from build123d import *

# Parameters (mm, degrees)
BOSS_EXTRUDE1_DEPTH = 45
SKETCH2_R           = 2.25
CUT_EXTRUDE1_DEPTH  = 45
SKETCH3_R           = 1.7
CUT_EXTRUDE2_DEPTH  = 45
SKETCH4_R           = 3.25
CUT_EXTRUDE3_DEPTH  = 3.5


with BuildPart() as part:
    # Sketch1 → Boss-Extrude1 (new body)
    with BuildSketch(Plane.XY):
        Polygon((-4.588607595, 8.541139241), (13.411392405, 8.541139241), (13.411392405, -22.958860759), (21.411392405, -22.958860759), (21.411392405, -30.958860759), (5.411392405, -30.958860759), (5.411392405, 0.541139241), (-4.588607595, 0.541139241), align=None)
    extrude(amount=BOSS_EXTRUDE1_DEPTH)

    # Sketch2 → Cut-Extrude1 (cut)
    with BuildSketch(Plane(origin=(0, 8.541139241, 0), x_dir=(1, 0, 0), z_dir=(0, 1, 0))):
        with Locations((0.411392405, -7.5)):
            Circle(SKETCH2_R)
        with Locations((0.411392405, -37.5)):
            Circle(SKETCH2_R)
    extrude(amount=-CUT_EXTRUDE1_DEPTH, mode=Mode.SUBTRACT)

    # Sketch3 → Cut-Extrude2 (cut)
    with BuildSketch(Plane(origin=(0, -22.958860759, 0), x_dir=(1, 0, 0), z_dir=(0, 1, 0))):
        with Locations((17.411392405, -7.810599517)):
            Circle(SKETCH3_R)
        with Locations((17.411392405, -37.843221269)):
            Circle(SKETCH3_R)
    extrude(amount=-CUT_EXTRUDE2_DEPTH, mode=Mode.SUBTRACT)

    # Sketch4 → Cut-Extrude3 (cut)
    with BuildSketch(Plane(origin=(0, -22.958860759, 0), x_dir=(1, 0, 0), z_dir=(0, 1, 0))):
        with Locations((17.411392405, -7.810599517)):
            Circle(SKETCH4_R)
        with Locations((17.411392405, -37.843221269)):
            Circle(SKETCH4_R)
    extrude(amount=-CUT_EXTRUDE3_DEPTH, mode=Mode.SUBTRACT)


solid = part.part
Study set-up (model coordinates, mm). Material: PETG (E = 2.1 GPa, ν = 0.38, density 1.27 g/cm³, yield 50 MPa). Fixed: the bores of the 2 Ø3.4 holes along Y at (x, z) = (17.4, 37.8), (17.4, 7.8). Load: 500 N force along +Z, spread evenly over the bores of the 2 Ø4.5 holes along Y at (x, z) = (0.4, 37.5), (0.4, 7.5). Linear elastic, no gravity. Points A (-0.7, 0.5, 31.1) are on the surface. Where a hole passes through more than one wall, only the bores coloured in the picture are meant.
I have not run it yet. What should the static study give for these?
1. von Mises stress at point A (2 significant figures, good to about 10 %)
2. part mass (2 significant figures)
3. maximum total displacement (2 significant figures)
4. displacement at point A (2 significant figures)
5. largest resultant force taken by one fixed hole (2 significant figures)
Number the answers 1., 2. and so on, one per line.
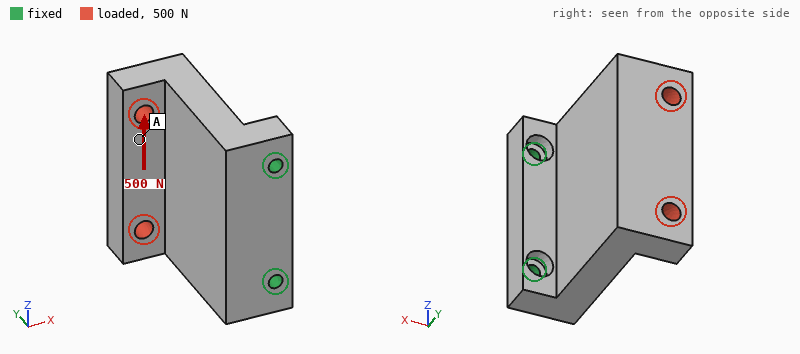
1. 4.0 MPa
2. 26 g
3. 0.54 mm
4. 0.39 mm
5. 640 N
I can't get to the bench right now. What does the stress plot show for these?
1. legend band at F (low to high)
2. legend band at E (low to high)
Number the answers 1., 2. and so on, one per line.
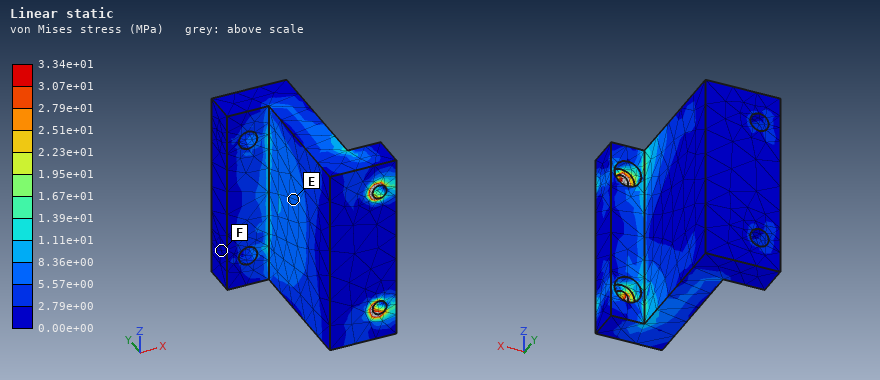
1. 0.00e+00 to 2.79e+00 MPa
2. 5.57e+00 to 8.36e+00 MPa
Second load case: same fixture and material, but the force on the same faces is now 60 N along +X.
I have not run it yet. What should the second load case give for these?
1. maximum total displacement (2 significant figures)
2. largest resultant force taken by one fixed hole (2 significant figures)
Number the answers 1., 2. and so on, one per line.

1. 0.71 mm
2. 38 N
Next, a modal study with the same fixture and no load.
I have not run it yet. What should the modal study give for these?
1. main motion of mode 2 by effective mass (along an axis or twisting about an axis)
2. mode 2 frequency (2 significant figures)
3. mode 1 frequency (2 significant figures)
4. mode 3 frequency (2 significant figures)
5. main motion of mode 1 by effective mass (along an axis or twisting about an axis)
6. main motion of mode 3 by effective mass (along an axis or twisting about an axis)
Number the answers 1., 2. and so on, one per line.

1. along Z
2. 1500 Hz
3. 480 Hz
4. 1800 Hz
5. along X
6. along Z
